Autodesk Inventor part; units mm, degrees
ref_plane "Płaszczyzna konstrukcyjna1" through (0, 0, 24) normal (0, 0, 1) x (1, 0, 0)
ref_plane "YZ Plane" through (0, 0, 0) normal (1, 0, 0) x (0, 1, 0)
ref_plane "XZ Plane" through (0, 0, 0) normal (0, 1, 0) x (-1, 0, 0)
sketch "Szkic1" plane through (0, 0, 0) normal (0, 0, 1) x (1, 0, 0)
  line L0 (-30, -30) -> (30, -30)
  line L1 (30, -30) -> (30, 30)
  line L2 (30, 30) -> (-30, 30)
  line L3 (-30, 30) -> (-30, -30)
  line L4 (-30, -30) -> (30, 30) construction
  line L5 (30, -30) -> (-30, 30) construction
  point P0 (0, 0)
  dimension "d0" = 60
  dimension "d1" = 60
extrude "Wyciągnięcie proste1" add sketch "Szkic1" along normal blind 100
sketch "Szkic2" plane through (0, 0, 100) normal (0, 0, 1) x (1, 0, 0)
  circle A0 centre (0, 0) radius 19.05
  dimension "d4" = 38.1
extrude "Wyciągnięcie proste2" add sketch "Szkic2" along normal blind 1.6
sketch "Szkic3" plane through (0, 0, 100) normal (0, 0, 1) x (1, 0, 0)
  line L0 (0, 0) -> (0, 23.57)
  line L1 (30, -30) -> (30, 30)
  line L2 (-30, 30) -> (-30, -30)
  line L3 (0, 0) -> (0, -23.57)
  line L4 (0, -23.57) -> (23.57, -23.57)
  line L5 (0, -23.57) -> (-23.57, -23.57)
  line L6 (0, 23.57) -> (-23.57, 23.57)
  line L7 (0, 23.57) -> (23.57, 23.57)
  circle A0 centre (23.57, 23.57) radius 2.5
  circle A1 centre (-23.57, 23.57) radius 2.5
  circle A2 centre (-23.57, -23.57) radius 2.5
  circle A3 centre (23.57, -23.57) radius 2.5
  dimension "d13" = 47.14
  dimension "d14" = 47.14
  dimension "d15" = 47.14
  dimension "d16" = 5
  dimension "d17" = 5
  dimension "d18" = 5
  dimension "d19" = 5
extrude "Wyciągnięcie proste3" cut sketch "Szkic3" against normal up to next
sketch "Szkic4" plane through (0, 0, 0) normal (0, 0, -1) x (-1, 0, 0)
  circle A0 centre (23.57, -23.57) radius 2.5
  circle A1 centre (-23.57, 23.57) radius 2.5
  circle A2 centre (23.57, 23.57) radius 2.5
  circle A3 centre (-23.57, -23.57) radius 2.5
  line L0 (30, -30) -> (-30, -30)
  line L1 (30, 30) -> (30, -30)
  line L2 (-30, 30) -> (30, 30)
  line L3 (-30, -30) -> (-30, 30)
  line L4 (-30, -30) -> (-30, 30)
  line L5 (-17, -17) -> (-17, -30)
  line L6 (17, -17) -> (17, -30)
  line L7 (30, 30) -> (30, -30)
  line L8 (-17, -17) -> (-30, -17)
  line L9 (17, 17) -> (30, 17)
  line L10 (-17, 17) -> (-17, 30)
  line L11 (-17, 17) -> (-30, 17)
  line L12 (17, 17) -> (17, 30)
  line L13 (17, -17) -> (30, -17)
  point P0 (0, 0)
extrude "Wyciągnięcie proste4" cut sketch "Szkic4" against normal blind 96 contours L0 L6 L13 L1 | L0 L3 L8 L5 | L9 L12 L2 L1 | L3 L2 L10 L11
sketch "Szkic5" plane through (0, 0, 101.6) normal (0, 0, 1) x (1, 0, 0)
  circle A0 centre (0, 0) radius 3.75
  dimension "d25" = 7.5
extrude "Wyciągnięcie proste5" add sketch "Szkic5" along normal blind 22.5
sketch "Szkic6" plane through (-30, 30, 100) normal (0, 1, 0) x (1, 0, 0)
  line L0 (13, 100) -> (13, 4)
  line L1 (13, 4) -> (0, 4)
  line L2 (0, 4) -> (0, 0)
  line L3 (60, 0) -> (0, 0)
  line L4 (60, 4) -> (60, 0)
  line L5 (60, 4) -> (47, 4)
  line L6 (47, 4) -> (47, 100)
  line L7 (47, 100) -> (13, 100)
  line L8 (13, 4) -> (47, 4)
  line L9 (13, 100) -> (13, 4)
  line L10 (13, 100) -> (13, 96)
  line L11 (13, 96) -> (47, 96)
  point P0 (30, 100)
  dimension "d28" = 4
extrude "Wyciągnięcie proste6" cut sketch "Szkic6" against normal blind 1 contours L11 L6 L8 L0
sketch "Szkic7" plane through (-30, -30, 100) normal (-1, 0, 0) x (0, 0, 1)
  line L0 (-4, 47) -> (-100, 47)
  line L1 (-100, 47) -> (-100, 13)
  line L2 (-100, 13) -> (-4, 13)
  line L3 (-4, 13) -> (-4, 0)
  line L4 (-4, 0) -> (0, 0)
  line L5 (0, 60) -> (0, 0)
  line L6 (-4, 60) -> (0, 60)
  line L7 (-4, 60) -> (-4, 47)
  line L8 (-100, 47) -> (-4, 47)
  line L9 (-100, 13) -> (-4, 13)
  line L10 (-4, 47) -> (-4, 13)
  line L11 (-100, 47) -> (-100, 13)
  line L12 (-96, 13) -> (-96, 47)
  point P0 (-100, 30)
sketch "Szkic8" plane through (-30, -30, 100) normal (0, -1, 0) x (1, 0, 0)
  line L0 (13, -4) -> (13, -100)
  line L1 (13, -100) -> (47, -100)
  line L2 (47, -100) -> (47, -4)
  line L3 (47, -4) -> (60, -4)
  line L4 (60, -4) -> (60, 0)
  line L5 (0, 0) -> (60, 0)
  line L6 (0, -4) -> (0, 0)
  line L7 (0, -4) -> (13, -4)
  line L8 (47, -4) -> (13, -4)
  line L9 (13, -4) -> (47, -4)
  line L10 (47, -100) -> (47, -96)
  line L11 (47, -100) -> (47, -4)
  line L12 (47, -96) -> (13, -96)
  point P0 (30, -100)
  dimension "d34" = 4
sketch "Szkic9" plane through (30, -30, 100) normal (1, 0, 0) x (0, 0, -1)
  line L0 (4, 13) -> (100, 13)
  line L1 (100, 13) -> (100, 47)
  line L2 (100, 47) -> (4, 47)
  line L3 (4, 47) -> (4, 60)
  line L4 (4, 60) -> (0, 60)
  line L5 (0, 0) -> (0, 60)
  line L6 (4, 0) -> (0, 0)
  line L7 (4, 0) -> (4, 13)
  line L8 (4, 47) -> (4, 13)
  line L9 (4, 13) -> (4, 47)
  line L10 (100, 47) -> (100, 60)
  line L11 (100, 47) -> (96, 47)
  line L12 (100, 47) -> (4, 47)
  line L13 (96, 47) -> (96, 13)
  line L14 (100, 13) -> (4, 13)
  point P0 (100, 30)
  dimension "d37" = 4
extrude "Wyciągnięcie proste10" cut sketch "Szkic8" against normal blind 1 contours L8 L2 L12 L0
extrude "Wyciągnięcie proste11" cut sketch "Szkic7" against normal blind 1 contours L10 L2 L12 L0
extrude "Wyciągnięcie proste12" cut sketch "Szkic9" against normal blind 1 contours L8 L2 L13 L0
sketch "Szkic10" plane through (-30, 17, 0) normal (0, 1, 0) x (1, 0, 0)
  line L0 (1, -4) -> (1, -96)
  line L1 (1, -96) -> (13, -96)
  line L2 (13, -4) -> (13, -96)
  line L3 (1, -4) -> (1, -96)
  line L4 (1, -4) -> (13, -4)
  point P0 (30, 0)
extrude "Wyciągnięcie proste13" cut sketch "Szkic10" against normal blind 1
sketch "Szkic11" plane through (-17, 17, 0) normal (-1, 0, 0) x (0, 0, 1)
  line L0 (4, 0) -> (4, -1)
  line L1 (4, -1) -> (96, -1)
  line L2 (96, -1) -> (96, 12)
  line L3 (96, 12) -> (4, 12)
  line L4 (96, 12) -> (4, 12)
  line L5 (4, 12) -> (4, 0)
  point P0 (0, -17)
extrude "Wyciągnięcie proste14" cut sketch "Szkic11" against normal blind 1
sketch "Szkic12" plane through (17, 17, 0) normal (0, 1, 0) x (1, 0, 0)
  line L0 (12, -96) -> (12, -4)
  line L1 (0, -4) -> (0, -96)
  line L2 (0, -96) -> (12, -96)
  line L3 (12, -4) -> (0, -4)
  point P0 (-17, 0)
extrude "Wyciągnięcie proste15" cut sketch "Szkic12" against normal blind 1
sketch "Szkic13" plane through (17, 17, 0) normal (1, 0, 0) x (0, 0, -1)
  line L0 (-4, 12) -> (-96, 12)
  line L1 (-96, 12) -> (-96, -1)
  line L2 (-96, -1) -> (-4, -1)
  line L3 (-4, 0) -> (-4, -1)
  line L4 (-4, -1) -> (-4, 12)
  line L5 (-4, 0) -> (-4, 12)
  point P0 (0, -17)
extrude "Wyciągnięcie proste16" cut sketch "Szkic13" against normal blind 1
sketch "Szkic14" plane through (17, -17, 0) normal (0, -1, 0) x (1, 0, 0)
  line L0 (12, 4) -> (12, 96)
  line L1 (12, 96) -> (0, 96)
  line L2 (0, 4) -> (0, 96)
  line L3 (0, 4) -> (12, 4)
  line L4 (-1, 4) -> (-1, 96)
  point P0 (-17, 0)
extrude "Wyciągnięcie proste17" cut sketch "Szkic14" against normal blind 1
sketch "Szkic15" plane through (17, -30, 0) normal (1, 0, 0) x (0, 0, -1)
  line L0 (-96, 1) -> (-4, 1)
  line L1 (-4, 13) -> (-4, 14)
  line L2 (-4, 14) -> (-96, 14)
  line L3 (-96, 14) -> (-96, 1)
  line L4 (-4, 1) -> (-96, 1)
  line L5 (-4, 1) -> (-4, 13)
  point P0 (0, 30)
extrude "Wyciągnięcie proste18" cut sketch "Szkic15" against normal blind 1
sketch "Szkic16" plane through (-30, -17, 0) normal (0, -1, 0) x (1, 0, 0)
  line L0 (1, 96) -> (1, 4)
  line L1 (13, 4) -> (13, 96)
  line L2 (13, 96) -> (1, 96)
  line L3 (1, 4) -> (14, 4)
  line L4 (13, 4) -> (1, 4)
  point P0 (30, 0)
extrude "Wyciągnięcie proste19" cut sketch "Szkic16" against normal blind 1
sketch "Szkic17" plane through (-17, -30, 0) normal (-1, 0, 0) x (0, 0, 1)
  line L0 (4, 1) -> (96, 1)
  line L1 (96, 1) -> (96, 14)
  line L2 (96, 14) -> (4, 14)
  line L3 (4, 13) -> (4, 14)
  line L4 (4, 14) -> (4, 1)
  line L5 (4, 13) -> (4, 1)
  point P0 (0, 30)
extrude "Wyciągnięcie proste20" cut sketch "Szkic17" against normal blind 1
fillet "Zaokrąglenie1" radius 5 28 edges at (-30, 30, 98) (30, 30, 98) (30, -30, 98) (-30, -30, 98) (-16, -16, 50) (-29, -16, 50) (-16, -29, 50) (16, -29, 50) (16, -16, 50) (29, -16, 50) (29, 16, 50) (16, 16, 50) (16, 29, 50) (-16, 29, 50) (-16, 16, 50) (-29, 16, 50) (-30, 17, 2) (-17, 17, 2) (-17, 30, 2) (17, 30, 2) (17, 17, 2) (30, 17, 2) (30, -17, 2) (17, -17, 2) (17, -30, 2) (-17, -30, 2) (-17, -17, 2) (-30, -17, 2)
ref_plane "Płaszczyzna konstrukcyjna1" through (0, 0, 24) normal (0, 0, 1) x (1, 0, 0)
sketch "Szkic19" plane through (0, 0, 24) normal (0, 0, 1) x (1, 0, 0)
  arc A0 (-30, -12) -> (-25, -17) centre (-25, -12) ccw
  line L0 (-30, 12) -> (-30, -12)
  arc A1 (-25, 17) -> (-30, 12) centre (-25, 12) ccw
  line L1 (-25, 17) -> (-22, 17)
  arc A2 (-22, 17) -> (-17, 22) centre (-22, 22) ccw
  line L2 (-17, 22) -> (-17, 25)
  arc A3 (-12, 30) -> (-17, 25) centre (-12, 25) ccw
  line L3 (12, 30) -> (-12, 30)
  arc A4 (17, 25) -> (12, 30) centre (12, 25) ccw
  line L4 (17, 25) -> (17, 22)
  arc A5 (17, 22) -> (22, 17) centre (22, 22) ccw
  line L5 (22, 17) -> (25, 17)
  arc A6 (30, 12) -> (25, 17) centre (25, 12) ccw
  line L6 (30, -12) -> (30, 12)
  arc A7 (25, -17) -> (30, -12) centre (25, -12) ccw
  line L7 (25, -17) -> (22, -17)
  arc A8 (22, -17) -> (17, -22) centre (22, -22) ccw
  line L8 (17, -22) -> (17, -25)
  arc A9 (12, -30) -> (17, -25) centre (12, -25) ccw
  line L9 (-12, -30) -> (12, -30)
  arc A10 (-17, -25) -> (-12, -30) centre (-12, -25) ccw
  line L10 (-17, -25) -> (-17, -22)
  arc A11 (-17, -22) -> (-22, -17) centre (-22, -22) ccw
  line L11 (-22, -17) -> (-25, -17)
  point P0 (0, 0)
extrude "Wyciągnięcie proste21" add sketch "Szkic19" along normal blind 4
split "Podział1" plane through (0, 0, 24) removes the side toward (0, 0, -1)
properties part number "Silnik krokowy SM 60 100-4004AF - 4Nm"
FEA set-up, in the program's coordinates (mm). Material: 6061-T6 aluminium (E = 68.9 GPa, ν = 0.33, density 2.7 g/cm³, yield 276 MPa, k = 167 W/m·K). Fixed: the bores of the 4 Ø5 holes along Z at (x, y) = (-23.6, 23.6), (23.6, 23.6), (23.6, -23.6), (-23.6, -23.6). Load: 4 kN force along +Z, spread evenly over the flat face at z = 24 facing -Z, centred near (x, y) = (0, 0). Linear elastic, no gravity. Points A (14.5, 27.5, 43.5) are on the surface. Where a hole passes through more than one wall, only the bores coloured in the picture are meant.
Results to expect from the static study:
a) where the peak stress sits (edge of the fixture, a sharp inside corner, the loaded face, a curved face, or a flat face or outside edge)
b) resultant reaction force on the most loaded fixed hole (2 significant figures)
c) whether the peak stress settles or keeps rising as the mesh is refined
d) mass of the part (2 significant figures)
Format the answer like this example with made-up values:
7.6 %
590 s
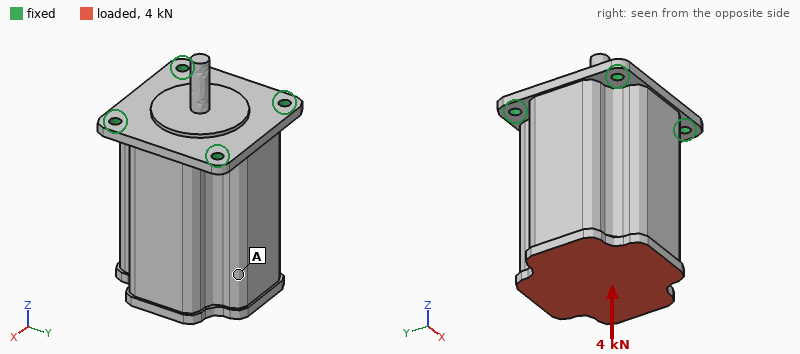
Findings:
edge of the fixture
1.1 kN
keeps rising
570 g
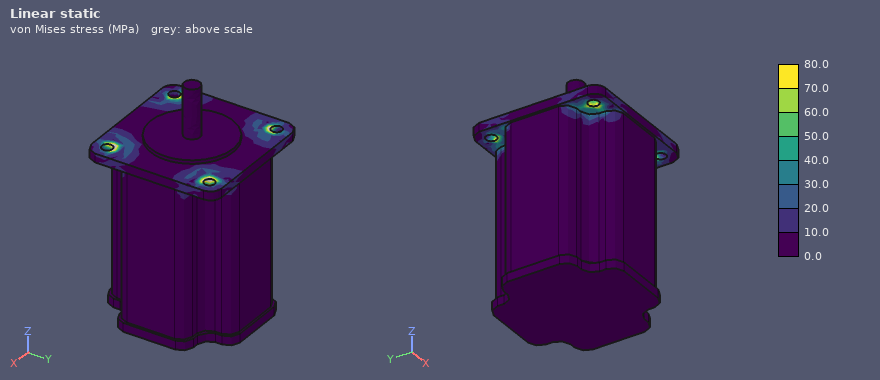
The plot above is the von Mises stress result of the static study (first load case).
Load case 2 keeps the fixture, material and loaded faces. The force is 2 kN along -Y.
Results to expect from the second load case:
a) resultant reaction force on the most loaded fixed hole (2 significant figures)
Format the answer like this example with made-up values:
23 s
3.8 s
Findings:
1.9 kN
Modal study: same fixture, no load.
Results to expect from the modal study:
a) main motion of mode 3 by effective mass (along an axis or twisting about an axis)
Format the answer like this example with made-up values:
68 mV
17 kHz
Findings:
along Z
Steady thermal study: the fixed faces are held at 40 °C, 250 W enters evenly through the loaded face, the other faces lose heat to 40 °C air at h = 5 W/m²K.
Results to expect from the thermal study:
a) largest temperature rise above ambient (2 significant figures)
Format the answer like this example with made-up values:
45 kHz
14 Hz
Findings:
83 K
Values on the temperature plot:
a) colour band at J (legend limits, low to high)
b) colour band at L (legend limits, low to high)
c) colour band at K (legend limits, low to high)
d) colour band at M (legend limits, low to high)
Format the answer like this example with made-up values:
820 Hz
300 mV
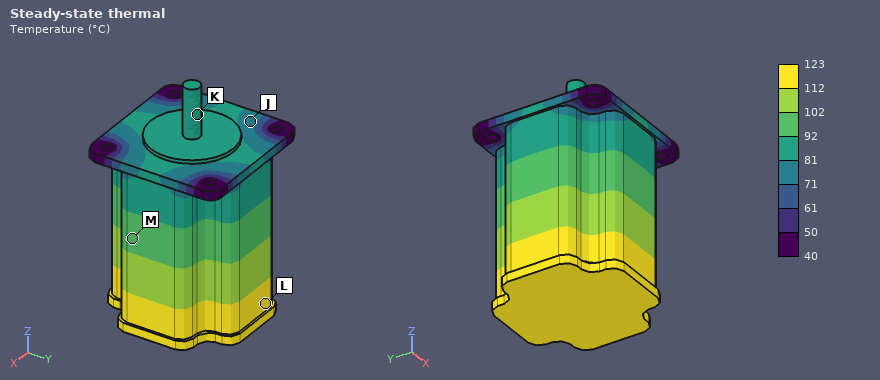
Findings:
71 to 81 °C
112 to 123 °C
81 to 92 °C
92 to 102 °C
